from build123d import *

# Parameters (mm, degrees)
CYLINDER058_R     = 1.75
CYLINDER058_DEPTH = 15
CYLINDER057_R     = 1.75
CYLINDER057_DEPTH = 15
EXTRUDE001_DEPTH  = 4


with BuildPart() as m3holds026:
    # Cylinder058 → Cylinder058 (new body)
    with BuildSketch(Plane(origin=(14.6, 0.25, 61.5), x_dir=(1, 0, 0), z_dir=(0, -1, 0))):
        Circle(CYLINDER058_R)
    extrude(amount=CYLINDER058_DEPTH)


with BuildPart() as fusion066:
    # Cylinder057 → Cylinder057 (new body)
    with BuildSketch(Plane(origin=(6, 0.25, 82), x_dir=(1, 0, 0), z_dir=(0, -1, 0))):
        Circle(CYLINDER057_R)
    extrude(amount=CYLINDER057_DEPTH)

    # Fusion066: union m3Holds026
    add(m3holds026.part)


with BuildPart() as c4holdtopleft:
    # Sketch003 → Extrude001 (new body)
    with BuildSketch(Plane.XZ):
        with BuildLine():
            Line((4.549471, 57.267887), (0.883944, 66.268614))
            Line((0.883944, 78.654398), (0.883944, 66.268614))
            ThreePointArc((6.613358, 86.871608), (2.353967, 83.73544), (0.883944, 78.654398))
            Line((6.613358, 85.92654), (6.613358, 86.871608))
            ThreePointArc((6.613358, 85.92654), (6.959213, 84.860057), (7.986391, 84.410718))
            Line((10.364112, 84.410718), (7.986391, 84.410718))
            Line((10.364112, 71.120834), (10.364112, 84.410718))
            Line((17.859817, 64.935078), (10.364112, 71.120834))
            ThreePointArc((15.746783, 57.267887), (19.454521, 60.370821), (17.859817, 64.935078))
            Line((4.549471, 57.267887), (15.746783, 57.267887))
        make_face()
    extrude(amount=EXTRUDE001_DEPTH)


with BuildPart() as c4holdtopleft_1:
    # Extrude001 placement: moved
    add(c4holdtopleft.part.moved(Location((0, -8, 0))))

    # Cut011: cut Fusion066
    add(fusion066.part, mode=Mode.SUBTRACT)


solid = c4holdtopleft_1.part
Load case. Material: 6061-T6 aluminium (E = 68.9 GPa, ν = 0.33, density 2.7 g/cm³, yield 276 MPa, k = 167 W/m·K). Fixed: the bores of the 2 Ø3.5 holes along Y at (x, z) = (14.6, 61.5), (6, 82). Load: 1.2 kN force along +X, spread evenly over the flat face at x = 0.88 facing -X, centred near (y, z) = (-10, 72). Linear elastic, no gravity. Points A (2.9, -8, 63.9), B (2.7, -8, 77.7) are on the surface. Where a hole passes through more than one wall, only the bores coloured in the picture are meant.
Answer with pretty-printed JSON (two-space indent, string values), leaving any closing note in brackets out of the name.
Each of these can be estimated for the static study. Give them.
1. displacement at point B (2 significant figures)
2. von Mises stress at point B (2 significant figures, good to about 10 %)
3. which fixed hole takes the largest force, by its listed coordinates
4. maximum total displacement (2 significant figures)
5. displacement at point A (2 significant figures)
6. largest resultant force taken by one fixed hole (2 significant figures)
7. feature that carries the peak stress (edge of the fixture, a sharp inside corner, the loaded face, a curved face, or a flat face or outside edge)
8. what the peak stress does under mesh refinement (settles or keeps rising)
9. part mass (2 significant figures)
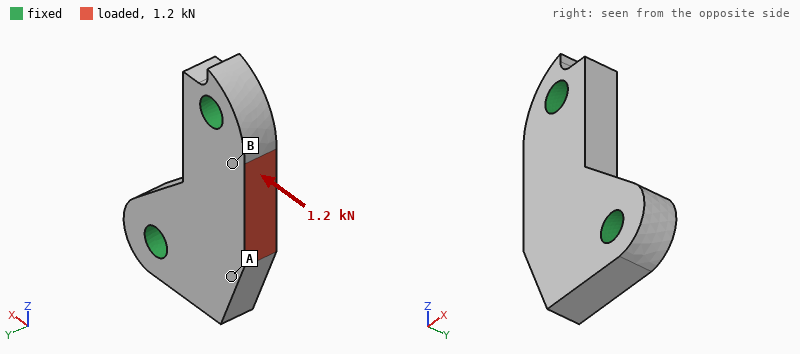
{
  "displacement at point B": "3.6 µm",
  "von Mises stress at point B": "30 MPa",
  "which fixed hole takes the largest force, by its listed coordinates": "(14.6, 61.5)",
  "maximum total displacement": "6.9 µm",
  "displacement at point A": "3.0 µm",
  "largest resultant force taken by one fixed hole": "740 N",
  "feature that carries the peak stress": "edge of the fixture",
  "what the peak stress does under mesh refinement": "keeps rising",
  "part mass": "3.4 g"
}
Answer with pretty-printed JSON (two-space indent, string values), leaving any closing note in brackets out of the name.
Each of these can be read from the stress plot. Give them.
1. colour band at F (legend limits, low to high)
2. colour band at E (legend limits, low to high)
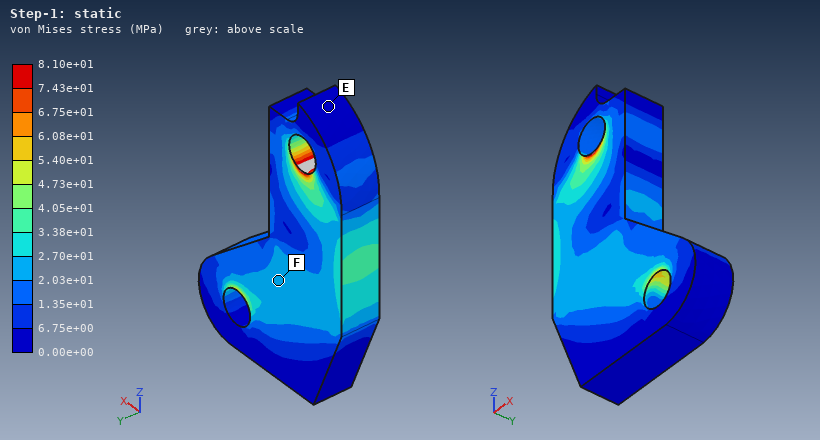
{
  "colour band at F": "2.03e+01 to 2.70e+01 MPa",
  "colour band at E": "0.00e+00 to 6.75e+00 MPa"
}
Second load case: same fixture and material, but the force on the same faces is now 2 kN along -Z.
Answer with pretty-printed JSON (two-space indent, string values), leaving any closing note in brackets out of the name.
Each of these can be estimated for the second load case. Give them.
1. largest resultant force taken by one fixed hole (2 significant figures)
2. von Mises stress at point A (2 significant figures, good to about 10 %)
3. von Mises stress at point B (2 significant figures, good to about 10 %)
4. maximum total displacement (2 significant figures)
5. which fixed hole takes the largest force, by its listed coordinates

{
  "largest resultant force taken by one fixed hole": "1.7 kN",
  "von Mises stress at point A": "27 MPa",
  "von Mises stress at point B": "67 MPa",
  "maximum total displacement": "10 µm",
  "which fixed hole takes the largest force, by its listed coordinates": "(6, 82)"
}
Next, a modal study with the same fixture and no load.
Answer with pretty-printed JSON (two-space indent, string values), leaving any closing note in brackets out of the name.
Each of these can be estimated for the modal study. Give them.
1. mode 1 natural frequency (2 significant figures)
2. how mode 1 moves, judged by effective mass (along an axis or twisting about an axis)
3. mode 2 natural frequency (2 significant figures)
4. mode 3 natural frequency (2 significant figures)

{
  "mode 1 natural frequency": "24 kHz",
  "how mode 1 moves, judged by effective mass": "along Y",
  "mode 2 natural frequency": "46 kHz",
  "mode 3 natural frequency": "55 kHz"
}
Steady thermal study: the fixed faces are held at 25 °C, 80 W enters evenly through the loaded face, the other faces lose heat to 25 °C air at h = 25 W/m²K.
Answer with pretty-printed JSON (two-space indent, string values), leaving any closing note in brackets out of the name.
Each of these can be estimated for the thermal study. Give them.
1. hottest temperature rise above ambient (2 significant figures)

{
  "hottest temperature rise above ambient": "81 K"
}
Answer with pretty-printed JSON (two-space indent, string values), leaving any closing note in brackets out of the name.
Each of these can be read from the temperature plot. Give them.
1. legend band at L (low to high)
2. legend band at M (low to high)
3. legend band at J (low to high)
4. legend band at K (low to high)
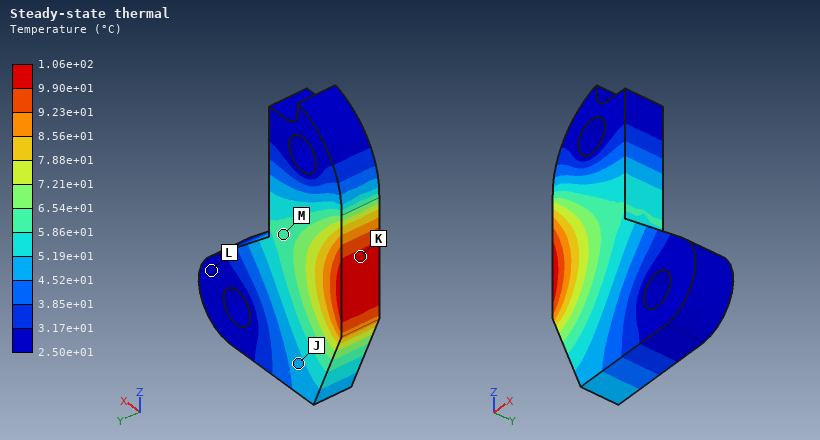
{
  "legend band at L": "2.50e+01 to 3.17e+01 °C",
  "legend band at M": "5.86e+01 to 6.54e+01 °C",
  "legend band at J": "4.52e+01 to 5.19e+01 °C",
  "legend band at K": "9.90e+01 to 1.06e+02 °C"
}
